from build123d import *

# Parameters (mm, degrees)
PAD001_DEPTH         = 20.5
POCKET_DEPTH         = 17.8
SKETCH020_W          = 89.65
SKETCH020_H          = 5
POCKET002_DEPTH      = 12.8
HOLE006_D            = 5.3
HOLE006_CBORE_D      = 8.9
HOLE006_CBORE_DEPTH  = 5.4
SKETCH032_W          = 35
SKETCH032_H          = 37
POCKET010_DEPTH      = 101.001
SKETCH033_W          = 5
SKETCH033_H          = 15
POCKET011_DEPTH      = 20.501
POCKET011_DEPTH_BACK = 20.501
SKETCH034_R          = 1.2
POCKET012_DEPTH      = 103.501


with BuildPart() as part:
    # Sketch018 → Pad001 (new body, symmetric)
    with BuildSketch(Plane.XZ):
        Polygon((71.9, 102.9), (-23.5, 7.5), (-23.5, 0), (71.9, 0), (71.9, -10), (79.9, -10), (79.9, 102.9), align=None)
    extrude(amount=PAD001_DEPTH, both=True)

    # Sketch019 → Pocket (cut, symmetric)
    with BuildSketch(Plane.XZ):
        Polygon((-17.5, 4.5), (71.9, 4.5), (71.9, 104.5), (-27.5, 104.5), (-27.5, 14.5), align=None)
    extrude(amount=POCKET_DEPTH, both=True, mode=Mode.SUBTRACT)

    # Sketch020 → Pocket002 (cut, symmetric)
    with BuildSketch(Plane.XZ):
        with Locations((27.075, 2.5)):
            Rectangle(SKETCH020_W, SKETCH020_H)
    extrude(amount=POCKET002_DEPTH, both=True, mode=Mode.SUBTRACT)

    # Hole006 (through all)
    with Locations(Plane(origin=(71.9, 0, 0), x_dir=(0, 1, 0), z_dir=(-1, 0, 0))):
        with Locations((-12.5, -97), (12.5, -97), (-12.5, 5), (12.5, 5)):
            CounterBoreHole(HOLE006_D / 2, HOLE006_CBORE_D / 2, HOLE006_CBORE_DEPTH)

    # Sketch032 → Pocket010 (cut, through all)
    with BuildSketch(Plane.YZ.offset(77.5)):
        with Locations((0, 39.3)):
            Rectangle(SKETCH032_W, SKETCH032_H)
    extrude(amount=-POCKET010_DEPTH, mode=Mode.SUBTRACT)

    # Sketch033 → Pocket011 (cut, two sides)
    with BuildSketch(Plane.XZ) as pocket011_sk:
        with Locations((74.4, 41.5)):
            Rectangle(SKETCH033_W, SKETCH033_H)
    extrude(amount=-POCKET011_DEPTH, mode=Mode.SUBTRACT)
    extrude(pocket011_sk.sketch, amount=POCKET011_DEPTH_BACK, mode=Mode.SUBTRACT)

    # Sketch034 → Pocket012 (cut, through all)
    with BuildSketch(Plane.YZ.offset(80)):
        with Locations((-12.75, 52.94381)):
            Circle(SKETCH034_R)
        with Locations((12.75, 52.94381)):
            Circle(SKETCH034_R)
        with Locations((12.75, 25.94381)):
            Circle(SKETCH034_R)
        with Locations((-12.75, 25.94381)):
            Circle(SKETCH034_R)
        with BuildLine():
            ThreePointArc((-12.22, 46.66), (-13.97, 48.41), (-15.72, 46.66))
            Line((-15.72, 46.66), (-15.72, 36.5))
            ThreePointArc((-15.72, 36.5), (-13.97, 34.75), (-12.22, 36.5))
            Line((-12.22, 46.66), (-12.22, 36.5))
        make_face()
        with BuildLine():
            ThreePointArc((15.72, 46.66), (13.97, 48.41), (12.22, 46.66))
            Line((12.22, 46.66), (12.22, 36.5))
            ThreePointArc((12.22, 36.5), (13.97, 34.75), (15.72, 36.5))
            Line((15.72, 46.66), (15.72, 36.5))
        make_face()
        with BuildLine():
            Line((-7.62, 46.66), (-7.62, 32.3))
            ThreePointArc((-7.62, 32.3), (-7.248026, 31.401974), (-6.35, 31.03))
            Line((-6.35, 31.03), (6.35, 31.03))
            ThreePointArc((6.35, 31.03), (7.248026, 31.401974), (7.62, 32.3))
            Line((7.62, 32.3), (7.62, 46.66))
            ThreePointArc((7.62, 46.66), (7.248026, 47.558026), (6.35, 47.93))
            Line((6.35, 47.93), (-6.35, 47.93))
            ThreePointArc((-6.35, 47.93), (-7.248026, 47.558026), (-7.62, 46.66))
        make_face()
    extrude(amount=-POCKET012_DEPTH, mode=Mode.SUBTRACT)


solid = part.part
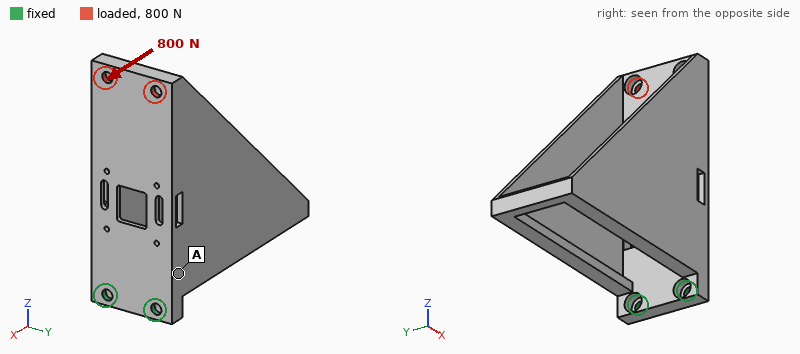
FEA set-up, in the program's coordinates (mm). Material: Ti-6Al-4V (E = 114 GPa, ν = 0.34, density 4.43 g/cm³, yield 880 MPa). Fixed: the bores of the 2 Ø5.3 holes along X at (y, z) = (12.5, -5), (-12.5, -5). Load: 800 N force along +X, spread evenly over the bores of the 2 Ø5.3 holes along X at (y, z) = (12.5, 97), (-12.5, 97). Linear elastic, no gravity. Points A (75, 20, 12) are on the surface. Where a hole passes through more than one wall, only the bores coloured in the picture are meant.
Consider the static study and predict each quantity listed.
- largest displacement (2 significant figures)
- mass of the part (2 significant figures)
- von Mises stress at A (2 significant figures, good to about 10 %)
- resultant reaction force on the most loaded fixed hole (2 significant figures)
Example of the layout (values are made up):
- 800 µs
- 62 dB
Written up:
- 1.7 mm
- 270 g
- 62 MPa
- 650 N
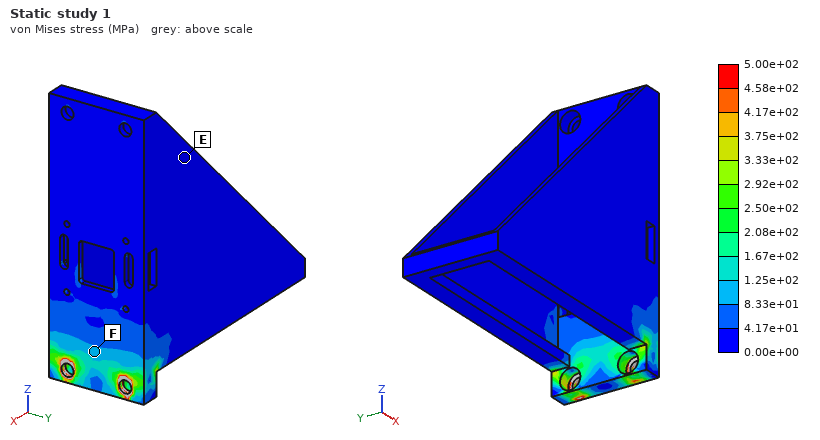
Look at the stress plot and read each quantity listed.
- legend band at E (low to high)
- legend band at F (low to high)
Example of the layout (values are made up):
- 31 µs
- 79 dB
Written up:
- 0.00e+00 to 4.17e+01 MPa
- 8.33e+01 to 1.25e+02 MPa
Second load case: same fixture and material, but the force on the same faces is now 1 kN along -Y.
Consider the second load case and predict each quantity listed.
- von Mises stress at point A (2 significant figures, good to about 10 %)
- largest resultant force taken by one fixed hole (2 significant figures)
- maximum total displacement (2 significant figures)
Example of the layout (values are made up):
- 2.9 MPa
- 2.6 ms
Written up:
- 34 MPa
- 3.7 kN
- 0.19 mm
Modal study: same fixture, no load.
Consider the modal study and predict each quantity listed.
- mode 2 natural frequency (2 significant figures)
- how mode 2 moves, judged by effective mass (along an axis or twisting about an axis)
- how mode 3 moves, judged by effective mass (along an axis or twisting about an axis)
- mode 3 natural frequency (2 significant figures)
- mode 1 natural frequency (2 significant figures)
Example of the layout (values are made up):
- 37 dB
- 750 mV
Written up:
- 630 Hz
- along Y
- along Y
- 1300 Hz
- 340 Hz
